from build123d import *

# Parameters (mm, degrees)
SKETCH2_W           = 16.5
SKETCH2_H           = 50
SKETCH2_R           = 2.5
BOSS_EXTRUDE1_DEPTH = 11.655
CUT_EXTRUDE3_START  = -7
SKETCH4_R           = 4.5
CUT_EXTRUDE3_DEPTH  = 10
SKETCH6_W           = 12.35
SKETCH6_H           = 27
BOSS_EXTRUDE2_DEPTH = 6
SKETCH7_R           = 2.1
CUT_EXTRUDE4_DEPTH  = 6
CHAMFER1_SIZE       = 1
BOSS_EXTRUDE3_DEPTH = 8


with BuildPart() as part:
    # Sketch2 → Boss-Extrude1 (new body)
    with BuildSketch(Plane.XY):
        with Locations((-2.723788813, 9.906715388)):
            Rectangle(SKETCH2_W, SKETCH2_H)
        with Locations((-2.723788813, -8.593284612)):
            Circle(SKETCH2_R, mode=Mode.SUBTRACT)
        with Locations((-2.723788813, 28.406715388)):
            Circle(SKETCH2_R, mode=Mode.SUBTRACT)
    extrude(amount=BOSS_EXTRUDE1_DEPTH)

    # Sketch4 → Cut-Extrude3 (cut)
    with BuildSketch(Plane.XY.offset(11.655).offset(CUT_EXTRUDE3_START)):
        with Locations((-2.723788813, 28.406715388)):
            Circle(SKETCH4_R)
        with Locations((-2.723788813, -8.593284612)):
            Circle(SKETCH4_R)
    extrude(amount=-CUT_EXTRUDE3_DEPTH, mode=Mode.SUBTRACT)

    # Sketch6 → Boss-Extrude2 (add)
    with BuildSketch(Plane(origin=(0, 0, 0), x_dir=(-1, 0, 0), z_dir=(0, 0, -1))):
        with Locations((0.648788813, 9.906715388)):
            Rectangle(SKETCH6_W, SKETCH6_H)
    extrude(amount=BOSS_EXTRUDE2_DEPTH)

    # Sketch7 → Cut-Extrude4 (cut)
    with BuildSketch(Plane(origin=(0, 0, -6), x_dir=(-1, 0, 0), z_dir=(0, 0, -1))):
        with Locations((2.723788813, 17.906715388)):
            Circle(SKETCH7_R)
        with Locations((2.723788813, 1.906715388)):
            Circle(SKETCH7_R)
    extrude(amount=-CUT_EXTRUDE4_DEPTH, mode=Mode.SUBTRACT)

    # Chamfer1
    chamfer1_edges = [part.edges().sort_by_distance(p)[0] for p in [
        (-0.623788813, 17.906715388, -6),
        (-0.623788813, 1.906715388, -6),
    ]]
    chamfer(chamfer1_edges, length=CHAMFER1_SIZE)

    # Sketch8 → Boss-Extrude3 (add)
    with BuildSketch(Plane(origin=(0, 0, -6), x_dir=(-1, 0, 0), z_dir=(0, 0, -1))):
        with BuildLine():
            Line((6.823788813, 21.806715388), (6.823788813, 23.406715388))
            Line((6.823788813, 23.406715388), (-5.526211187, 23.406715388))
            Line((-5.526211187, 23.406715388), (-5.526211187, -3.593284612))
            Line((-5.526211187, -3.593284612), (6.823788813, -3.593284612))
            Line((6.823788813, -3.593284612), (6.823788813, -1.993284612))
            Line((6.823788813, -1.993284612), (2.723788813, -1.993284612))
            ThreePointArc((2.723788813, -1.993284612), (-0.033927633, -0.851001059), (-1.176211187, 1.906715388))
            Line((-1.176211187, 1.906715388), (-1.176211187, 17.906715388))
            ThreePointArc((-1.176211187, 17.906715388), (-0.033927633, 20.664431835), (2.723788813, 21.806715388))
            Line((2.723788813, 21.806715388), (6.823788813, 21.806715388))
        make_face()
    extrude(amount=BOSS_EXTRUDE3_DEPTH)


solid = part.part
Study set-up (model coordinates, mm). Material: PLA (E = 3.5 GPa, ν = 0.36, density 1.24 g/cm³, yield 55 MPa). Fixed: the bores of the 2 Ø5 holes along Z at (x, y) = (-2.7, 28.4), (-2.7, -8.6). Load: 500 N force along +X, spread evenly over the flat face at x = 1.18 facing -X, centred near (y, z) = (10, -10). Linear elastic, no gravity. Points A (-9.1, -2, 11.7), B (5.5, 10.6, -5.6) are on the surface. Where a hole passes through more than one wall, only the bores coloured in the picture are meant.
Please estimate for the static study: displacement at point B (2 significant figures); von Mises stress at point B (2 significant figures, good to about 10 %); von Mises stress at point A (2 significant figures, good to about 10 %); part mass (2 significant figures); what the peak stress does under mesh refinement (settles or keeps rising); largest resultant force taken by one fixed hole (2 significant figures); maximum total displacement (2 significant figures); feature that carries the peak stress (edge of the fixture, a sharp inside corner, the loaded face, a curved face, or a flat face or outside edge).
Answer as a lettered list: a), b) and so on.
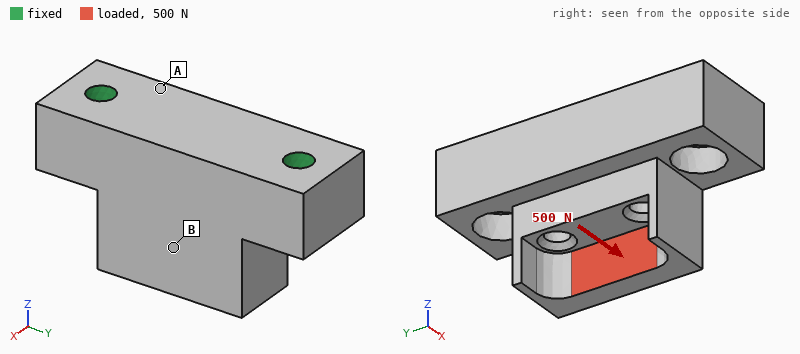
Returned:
a) 0.24 mm
b) 15 MPa
c) 5.5 MPa
d) 15 g
e) keeps rising
f) 250 N
g) 0.46 mm
h) edge of the fixture
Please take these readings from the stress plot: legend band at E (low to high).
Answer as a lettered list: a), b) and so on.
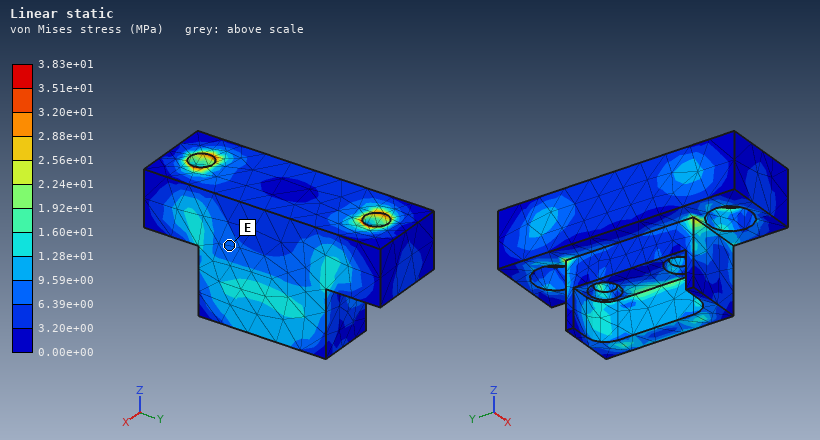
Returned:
a) 6.39e+00 to 9.59e+00 MPa
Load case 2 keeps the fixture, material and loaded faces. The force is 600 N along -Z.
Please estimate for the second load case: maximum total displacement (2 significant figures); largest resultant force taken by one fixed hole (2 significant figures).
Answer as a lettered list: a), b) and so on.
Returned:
a) 80 µm
b) 340 N
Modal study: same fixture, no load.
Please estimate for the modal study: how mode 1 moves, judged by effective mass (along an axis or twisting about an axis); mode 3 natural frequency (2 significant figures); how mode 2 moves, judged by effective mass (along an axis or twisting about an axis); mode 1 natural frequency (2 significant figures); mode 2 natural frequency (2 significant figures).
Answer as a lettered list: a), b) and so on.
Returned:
a) along X
b) 8800 Hz
c) along Z
d) 3900 Hz
e) 7800 Hz
